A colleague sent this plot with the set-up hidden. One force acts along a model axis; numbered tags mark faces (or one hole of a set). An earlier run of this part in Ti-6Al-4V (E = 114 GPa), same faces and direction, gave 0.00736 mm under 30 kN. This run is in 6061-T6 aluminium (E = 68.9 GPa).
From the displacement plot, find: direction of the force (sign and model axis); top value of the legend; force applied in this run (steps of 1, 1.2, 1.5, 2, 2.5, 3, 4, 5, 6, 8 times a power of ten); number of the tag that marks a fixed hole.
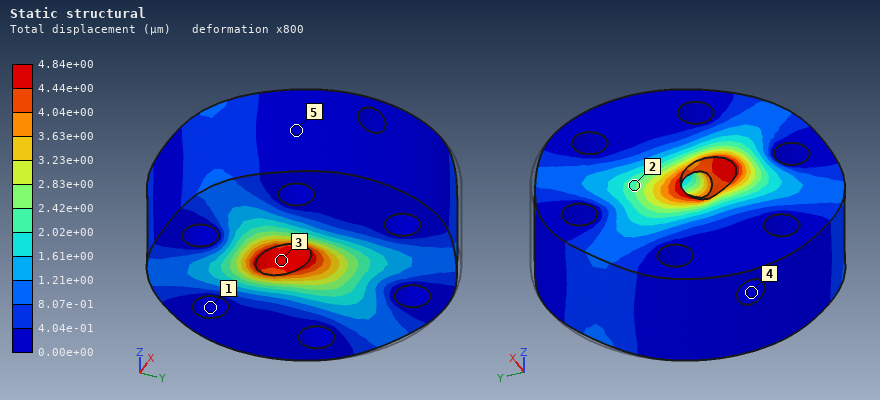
-Y
4.84e+00 µm
12 kN
1
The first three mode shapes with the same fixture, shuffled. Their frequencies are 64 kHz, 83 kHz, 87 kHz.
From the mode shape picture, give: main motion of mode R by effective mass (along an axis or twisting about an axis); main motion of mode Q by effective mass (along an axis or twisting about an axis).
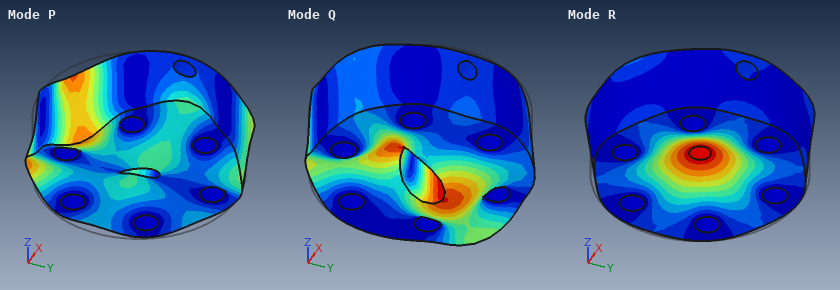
along Z
twisting about X
